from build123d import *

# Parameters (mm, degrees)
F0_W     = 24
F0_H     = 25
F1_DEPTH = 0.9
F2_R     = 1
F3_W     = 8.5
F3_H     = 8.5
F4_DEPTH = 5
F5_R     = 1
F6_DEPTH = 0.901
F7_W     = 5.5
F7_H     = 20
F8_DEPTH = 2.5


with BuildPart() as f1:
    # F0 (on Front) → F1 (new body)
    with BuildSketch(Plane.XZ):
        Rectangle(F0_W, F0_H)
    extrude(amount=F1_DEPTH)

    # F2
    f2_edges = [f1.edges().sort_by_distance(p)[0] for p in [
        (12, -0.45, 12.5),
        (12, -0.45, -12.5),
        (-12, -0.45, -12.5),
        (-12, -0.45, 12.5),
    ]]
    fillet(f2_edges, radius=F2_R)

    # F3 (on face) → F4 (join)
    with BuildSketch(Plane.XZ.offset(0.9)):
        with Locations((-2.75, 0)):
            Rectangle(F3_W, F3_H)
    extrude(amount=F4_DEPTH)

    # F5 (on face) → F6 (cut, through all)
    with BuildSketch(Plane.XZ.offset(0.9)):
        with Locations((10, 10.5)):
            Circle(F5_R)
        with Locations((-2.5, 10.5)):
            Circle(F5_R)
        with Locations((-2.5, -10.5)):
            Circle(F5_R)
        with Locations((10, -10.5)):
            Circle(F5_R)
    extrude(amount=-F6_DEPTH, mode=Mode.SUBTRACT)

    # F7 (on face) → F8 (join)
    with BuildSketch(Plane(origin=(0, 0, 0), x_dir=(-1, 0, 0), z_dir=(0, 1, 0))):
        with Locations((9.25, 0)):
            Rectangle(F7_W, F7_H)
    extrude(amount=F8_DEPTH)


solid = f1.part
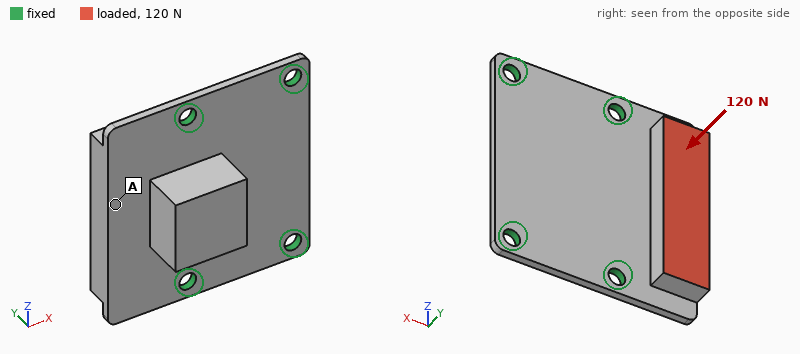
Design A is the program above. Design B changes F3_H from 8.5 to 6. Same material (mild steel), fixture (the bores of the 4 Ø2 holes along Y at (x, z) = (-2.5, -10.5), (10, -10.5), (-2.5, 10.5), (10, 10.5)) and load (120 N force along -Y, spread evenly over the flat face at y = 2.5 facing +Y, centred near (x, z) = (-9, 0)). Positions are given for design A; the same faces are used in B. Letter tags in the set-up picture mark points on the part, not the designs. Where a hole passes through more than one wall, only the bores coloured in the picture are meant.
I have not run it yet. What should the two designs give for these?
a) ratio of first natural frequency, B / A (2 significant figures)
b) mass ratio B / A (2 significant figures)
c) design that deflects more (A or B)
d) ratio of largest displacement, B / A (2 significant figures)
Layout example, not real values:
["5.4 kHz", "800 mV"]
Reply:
["0.97", "0.91", "B", "1.1"]
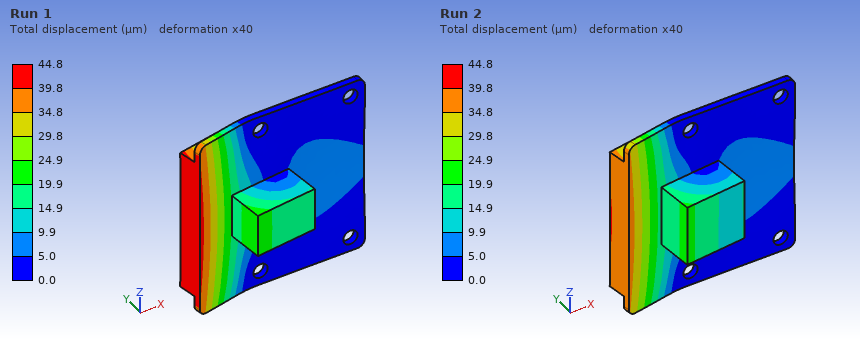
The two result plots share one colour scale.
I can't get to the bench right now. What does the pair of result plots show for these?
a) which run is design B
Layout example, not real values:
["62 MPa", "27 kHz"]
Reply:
["Run 1"]
